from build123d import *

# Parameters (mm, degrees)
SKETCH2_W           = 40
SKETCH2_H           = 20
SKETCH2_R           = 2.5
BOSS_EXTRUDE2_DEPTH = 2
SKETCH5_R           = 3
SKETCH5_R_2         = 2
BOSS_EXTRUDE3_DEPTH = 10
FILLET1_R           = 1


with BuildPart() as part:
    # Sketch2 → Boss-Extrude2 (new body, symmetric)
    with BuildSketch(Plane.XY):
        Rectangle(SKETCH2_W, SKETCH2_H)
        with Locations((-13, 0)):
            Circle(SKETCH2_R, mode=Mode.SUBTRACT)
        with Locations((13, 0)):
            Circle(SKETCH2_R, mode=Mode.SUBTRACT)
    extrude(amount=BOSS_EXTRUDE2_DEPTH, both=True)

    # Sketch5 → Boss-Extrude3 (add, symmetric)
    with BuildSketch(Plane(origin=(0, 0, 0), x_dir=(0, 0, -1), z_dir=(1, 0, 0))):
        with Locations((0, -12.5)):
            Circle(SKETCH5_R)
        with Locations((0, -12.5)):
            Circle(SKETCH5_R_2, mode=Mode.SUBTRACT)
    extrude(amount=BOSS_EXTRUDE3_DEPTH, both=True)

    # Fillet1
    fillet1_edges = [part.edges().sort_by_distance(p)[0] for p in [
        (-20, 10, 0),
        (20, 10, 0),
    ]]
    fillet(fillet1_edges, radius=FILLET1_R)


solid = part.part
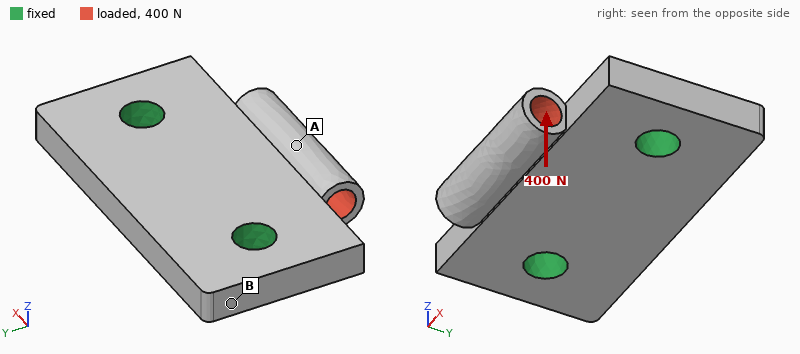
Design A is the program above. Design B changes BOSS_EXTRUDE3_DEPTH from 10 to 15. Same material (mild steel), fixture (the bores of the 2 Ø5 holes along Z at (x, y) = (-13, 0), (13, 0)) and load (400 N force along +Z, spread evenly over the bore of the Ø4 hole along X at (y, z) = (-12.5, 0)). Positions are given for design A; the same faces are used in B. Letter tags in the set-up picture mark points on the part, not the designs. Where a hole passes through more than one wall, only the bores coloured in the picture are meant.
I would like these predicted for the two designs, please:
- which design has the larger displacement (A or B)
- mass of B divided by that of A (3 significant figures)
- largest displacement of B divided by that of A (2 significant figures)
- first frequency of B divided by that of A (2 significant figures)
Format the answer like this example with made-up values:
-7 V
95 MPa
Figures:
A
1.04
0.74
0.97
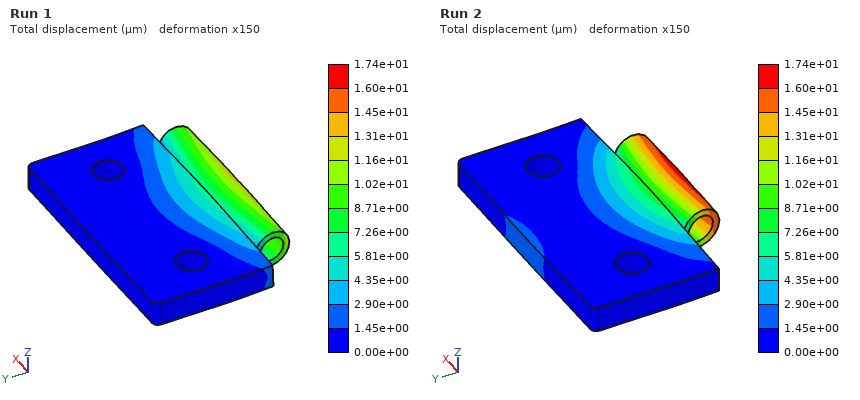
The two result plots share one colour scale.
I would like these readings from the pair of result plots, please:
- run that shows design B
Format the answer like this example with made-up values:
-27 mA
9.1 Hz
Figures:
Run 1
